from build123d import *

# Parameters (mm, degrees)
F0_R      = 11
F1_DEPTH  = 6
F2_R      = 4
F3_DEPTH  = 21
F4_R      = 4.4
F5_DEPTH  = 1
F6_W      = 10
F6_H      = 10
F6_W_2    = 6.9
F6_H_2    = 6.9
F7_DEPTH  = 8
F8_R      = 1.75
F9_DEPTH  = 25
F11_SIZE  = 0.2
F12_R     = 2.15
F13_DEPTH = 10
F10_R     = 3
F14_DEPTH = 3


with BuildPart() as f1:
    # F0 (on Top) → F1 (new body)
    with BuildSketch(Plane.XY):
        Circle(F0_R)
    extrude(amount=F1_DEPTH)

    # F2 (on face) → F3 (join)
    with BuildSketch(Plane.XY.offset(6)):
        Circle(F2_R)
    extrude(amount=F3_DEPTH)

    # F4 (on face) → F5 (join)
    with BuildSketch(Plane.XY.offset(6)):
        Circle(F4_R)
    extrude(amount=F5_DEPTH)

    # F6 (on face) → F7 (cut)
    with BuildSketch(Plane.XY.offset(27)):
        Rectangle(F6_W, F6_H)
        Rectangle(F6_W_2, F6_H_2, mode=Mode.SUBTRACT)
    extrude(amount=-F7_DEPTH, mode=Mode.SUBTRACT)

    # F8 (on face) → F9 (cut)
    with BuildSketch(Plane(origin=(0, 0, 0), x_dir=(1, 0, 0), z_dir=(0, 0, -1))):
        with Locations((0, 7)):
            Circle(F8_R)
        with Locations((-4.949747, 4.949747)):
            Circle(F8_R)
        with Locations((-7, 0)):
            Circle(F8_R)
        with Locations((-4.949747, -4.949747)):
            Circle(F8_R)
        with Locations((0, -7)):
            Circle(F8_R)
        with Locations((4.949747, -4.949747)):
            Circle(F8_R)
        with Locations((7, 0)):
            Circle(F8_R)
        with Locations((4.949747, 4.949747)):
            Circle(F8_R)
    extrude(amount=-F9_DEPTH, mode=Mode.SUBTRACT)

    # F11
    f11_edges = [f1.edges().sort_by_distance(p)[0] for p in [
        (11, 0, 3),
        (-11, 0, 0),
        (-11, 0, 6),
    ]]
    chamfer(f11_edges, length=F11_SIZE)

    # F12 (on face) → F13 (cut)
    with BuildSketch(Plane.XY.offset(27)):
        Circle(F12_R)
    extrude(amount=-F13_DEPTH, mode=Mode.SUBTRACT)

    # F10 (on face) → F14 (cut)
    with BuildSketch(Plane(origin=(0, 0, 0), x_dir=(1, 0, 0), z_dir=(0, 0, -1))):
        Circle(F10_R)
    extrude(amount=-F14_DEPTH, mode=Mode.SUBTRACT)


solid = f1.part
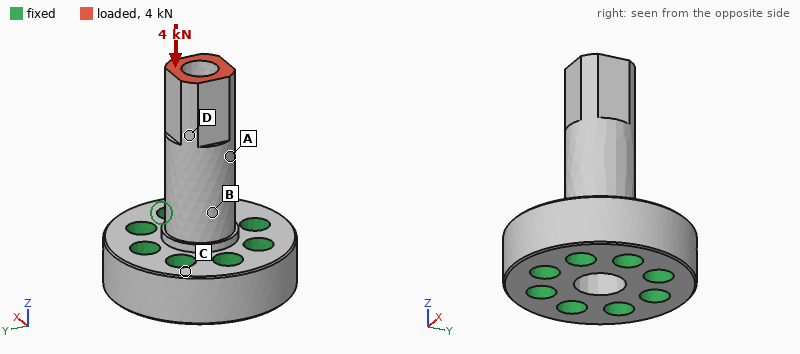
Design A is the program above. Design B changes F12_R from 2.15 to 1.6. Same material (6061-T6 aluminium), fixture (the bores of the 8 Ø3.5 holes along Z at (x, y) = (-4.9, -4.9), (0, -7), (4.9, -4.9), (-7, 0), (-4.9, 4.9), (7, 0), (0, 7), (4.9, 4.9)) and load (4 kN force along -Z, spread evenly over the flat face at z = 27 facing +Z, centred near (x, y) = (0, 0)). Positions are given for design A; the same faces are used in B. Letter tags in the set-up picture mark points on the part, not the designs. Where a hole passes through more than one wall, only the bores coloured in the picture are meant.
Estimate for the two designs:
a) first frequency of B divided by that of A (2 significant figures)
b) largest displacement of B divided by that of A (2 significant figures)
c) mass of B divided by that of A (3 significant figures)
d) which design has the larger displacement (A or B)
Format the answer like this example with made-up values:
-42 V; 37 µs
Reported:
0.93; 0.89; 1.02; A
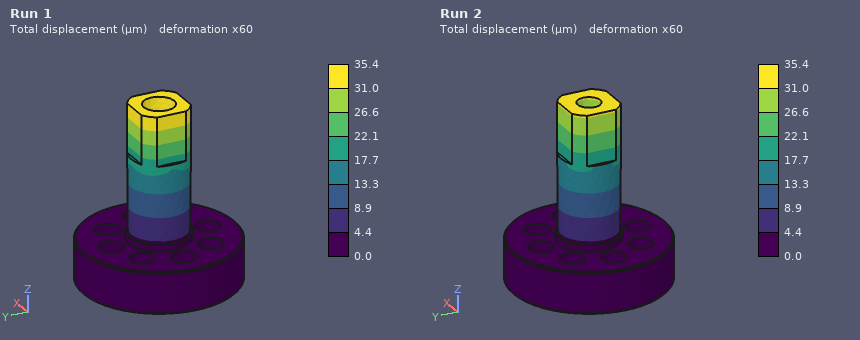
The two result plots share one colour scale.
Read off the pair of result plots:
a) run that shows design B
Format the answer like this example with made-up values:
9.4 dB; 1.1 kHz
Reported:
Run 2
